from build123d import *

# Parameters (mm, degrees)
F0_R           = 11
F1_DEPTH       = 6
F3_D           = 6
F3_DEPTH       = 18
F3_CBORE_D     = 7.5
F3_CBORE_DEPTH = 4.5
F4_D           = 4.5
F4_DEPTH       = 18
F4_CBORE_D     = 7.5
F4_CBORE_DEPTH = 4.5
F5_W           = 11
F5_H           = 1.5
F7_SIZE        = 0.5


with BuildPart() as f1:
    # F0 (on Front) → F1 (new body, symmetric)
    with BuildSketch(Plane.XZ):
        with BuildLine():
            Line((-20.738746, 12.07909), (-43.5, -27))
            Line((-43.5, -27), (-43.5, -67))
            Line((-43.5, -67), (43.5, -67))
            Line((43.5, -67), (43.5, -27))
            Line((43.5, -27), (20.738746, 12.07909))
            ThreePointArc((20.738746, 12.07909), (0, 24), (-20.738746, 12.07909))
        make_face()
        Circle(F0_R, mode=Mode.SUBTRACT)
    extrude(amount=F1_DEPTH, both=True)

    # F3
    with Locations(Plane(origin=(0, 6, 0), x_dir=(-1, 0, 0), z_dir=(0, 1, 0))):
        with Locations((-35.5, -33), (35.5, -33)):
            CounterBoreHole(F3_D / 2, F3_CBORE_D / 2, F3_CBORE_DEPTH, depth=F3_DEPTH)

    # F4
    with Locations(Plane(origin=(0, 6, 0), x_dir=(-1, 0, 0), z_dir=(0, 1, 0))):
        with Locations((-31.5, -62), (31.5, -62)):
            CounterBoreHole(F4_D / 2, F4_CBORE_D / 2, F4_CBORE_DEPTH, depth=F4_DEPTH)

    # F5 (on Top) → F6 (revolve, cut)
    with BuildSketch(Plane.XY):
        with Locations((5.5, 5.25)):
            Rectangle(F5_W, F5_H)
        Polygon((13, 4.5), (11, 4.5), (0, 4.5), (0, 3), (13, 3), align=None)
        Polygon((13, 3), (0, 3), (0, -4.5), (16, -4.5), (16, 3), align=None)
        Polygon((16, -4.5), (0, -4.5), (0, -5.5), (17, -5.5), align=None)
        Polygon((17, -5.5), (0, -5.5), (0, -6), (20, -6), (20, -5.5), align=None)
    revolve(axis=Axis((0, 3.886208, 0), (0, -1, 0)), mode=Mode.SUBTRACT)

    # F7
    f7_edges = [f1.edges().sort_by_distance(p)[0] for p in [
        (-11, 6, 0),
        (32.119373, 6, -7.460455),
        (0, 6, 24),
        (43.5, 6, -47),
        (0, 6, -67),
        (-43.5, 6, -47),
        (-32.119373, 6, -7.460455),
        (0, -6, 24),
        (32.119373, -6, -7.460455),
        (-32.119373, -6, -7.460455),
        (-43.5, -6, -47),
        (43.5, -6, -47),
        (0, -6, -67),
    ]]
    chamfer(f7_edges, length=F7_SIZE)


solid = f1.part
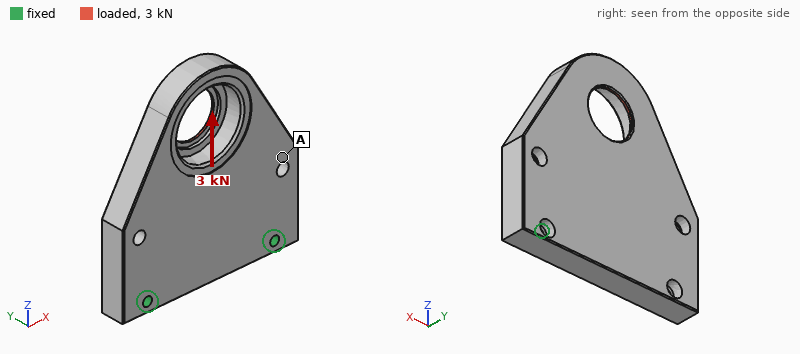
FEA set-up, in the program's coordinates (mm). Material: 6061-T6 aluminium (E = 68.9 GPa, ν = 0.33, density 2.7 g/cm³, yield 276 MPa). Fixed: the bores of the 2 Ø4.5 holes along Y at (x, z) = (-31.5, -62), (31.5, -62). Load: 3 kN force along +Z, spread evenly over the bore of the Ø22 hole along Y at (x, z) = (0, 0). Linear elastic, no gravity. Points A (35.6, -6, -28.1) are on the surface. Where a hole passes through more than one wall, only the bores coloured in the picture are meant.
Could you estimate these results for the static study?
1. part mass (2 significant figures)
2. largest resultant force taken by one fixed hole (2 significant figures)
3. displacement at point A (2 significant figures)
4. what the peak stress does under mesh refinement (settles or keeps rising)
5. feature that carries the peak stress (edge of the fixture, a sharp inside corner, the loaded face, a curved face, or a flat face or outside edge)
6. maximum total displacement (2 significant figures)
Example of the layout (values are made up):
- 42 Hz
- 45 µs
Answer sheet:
- 180 g
- 1.5 kN
- 0.038 mm
- keeps rising
- edge of the fixture
- 0.16 mm
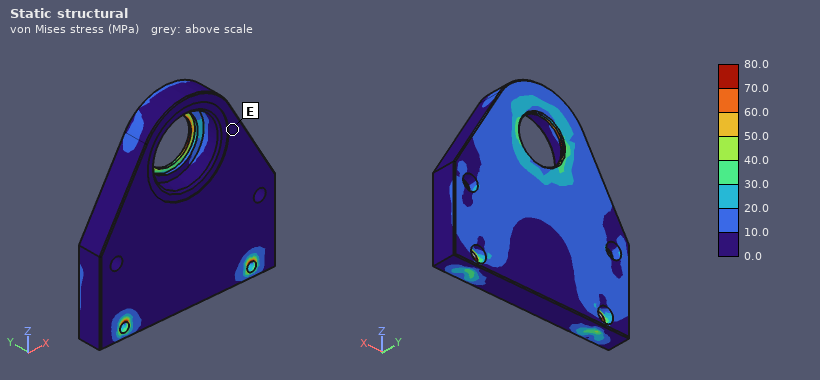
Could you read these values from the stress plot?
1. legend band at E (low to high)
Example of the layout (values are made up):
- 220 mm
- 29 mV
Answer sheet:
- 0.0 to 10.0 MPa
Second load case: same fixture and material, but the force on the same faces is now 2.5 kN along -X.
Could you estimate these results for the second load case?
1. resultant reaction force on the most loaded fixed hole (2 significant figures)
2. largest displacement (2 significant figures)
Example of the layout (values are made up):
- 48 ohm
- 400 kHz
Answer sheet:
- 2.7 kN
- 35 µm
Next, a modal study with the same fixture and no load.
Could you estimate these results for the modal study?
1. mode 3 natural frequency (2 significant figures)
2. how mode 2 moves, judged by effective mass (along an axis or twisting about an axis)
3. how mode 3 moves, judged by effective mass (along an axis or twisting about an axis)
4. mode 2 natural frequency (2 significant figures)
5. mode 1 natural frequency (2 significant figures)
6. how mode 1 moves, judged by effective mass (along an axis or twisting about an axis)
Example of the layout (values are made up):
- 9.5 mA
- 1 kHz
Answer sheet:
- 6100 Hz
- twisting about Z
- along Y
- 4300 Hz
- 1300 Hz
- along Y
